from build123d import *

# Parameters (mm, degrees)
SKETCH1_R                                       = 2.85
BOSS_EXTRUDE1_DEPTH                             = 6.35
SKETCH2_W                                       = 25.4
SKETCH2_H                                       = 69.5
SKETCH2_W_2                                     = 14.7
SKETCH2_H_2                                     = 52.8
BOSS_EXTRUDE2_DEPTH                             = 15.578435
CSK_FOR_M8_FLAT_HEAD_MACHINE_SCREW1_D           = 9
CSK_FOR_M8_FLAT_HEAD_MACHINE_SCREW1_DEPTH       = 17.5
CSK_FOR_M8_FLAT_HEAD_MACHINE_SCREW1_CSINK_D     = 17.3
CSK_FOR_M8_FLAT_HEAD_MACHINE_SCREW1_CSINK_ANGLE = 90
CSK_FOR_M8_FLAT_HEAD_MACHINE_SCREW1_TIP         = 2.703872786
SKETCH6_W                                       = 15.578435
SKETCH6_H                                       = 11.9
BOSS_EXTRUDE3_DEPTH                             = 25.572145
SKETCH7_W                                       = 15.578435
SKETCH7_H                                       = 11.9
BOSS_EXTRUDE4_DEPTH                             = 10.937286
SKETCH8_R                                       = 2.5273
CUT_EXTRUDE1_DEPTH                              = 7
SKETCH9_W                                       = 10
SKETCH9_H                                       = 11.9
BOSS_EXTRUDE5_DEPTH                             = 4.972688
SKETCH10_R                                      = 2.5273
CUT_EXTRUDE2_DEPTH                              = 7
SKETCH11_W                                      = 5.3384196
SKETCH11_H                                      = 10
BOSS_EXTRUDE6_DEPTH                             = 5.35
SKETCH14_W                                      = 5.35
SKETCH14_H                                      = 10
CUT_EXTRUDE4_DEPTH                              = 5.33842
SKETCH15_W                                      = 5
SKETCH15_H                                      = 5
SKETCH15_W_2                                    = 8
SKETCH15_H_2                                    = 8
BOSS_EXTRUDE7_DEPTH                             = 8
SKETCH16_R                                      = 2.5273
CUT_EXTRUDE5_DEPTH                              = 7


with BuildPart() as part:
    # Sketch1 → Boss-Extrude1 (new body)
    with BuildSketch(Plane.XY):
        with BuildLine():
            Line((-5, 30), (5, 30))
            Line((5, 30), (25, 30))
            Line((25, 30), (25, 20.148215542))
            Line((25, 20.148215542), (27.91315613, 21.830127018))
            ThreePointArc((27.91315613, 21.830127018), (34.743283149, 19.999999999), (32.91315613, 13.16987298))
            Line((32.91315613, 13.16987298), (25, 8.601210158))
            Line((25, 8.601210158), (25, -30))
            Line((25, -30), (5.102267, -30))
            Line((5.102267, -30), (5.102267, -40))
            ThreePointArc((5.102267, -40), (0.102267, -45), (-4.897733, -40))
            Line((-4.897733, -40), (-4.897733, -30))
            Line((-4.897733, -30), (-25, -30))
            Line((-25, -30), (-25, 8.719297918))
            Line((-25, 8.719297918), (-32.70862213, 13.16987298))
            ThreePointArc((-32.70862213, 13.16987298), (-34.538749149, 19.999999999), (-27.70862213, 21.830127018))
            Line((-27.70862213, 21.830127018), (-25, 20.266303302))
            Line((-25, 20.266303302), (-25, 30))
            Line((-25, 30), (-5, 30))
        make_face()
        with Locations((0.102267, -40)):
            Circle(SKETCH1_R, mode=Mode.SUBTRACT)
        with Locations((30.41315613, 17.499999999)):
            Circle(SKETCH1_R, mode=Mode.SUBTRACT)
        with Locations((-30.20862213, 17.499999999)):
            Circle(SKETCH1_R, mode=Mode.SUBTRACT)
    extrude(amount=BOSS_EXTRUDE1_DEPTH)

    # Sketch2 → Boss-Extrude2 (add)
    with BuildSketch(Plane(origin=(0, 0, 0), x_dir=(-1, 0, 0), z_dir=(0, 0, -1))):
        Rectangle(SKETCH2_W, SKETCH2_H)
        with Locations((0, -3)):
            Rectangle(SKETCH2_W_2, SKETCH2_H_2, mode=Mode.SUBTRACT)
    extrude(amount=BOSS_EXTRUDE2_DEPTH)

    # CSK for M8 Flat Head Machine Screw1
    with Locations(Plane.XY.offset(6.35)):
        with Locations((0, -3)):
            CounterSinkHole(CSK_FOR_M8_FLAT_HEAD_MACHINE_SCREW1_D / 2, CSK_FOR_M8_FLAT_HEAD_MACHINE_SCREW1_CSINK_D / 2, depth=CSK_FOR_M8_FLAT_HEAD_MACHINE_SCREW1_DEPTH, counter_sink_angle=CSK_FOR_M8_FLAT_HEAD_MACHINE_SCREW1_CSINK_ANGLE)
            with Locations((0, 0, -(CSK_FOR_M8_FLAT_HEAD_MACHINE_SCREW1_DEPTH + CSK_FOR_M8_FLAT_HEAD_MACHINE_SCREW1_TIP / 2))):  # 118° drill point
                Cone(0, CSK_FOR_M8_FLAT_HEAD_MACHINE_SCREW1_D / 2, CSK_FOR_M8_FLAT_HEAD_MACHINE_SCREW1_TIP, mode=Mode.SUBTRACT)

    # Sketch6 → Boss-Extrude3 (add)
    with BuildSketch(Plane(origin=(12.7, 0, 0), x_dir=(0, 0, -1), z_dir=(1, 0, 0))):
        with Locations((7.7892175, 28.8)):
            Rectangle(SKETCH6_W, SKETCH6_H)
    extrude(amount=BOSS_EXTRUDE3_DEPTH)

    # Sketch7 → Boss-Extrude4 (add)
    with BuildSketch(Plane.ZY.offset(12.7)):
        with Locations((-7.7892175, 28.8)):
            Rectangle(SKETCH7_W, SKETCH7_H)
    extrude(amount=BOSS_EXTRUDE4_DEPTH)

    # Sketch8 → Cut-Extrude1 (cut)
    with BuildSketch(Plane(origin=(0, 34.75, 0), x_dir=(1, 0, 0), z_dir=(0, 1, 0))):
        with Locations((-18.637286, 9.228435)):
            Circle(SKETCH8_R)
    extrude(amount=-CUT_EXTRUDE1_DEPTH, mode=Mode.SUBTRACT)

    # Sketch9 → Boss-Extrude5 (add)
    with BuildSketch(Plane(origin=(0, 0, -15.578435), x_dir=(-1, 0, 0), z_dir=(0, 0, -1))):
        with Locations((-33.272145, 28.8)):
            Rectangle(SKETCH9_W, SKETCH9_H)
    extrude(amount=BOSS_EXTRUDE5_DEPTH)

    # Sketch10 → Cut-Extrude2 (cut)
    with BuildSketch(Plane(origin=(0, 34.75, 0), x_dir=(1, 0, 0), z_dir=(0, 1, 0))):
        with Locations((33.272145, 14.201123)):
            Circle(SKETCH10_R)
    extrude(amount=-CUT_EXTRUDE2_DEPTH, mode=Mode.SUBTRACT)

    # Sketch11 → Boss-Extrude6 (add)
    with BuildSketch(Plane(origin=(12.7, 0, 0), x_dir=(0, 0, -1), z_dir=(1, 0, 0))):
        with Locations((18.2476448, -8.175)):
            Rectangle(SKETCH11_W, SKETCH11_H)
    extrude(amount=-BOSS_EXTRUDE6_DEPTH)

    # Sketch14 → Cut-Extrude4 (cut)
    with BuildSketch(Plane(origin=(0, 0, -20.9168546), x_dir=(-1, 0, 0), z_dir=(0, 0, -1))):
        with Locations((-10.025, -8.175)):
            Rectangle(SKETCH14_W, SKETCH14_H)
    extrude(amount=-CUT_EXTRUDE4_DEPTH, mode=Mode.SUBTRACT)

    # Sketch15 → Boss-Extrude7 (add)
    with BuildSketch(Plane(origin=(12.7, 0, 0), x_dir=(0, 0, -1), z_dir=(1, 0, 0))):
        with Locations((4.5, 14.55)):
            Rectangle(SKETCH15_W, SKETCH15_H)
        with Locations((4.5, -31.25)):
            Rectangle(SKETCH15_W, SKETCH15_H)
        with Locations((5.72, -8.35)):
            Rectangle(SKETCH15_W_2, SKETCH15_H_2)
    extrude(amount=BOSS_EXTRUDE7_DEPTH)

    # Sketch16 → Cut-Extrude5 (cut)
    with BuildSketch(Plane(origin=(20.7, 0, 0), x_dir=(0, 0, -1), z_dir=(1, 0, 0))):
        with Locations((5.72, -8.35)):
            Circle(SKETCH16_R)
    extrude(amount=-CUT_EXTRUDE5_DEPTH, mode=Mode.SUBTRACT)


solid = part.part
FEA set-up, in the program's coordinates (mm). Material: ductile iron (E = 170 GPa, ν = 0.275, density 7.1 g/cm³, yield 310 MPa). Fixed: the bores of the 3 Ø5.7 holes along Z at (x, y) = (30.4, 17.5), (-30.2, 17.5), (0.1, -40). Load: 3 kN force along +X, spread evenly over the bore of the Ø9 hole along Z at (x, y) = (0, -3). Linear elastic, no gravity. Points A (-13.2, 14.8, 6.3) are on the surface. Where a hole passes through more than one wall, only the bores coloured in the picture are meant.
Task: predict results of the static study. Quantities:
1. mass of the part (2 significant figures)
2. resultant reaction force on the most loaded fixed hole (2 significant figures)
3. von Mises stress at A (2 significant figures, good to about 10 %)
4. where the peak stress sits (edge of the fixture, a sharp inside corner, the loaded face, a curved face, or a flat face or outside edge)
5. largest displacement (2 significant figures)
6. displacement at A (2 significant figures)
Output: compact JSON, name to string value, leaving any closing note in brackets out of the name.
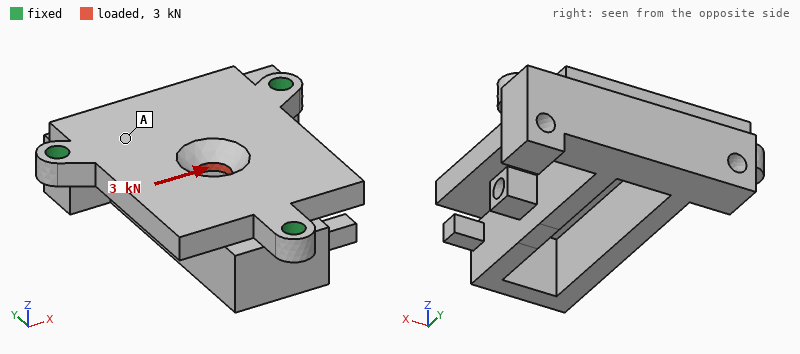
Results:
{"mass of the part": "310 g", "resultant reaction force on the most loaded fixed hole": "1.3 kN", "von Mises stress at A": "6.4 MPa", "where the peak stress sits": "the loaded face", "largest displacement": "4.8 µm", "displacement at A": "1.2 µm"}
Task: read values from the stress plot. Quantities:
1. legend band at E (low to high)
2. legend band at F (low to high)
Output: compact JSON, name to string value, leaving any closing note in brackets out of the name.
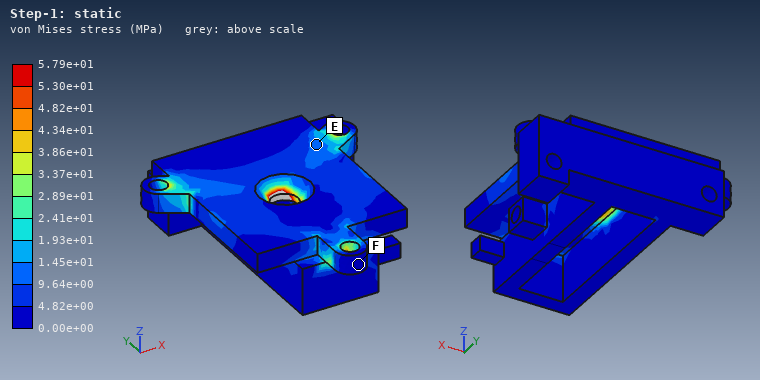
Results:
{"legend band at E": "9.64e+00 to 1.45e+01 MPa", "legend band at F": "0.00e+00 to 4.82e+00 MPa"}
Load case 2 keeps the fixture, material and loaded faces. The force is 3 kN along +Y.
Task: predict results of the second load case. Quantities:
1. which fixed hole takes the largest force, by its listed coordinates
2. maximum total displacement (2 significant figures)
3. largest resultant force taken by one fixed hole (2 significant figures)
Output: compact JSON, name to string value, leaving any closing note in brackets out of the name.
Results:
{"which fixed hole takes the largest force, by its listed coordinates": "(0.1, -40)", "maximum total displacement": "4.4 µm", "largest resultant force taken by one fixed hole": "1.4 kN"}
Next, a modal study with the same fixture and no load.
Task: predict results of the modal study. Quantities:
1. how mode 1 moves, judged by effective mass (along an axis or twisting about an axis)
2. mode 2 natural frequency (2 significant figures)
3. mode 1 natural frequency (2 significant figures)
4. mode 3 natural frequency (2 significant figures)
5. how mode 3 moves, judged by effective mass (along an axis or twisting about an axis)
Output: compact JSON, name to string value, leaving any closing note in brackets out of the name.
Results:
{"how mode 1 moves, judged by effective mass": "along Z", "mode 2 natural frequency": "5500 Hz", "mode 1 natural frequency": "5100 Hz", "mode 3 natural frequency": "7100 Hz", "how mode 3 moves, judged by effective mass": "along Z"}
